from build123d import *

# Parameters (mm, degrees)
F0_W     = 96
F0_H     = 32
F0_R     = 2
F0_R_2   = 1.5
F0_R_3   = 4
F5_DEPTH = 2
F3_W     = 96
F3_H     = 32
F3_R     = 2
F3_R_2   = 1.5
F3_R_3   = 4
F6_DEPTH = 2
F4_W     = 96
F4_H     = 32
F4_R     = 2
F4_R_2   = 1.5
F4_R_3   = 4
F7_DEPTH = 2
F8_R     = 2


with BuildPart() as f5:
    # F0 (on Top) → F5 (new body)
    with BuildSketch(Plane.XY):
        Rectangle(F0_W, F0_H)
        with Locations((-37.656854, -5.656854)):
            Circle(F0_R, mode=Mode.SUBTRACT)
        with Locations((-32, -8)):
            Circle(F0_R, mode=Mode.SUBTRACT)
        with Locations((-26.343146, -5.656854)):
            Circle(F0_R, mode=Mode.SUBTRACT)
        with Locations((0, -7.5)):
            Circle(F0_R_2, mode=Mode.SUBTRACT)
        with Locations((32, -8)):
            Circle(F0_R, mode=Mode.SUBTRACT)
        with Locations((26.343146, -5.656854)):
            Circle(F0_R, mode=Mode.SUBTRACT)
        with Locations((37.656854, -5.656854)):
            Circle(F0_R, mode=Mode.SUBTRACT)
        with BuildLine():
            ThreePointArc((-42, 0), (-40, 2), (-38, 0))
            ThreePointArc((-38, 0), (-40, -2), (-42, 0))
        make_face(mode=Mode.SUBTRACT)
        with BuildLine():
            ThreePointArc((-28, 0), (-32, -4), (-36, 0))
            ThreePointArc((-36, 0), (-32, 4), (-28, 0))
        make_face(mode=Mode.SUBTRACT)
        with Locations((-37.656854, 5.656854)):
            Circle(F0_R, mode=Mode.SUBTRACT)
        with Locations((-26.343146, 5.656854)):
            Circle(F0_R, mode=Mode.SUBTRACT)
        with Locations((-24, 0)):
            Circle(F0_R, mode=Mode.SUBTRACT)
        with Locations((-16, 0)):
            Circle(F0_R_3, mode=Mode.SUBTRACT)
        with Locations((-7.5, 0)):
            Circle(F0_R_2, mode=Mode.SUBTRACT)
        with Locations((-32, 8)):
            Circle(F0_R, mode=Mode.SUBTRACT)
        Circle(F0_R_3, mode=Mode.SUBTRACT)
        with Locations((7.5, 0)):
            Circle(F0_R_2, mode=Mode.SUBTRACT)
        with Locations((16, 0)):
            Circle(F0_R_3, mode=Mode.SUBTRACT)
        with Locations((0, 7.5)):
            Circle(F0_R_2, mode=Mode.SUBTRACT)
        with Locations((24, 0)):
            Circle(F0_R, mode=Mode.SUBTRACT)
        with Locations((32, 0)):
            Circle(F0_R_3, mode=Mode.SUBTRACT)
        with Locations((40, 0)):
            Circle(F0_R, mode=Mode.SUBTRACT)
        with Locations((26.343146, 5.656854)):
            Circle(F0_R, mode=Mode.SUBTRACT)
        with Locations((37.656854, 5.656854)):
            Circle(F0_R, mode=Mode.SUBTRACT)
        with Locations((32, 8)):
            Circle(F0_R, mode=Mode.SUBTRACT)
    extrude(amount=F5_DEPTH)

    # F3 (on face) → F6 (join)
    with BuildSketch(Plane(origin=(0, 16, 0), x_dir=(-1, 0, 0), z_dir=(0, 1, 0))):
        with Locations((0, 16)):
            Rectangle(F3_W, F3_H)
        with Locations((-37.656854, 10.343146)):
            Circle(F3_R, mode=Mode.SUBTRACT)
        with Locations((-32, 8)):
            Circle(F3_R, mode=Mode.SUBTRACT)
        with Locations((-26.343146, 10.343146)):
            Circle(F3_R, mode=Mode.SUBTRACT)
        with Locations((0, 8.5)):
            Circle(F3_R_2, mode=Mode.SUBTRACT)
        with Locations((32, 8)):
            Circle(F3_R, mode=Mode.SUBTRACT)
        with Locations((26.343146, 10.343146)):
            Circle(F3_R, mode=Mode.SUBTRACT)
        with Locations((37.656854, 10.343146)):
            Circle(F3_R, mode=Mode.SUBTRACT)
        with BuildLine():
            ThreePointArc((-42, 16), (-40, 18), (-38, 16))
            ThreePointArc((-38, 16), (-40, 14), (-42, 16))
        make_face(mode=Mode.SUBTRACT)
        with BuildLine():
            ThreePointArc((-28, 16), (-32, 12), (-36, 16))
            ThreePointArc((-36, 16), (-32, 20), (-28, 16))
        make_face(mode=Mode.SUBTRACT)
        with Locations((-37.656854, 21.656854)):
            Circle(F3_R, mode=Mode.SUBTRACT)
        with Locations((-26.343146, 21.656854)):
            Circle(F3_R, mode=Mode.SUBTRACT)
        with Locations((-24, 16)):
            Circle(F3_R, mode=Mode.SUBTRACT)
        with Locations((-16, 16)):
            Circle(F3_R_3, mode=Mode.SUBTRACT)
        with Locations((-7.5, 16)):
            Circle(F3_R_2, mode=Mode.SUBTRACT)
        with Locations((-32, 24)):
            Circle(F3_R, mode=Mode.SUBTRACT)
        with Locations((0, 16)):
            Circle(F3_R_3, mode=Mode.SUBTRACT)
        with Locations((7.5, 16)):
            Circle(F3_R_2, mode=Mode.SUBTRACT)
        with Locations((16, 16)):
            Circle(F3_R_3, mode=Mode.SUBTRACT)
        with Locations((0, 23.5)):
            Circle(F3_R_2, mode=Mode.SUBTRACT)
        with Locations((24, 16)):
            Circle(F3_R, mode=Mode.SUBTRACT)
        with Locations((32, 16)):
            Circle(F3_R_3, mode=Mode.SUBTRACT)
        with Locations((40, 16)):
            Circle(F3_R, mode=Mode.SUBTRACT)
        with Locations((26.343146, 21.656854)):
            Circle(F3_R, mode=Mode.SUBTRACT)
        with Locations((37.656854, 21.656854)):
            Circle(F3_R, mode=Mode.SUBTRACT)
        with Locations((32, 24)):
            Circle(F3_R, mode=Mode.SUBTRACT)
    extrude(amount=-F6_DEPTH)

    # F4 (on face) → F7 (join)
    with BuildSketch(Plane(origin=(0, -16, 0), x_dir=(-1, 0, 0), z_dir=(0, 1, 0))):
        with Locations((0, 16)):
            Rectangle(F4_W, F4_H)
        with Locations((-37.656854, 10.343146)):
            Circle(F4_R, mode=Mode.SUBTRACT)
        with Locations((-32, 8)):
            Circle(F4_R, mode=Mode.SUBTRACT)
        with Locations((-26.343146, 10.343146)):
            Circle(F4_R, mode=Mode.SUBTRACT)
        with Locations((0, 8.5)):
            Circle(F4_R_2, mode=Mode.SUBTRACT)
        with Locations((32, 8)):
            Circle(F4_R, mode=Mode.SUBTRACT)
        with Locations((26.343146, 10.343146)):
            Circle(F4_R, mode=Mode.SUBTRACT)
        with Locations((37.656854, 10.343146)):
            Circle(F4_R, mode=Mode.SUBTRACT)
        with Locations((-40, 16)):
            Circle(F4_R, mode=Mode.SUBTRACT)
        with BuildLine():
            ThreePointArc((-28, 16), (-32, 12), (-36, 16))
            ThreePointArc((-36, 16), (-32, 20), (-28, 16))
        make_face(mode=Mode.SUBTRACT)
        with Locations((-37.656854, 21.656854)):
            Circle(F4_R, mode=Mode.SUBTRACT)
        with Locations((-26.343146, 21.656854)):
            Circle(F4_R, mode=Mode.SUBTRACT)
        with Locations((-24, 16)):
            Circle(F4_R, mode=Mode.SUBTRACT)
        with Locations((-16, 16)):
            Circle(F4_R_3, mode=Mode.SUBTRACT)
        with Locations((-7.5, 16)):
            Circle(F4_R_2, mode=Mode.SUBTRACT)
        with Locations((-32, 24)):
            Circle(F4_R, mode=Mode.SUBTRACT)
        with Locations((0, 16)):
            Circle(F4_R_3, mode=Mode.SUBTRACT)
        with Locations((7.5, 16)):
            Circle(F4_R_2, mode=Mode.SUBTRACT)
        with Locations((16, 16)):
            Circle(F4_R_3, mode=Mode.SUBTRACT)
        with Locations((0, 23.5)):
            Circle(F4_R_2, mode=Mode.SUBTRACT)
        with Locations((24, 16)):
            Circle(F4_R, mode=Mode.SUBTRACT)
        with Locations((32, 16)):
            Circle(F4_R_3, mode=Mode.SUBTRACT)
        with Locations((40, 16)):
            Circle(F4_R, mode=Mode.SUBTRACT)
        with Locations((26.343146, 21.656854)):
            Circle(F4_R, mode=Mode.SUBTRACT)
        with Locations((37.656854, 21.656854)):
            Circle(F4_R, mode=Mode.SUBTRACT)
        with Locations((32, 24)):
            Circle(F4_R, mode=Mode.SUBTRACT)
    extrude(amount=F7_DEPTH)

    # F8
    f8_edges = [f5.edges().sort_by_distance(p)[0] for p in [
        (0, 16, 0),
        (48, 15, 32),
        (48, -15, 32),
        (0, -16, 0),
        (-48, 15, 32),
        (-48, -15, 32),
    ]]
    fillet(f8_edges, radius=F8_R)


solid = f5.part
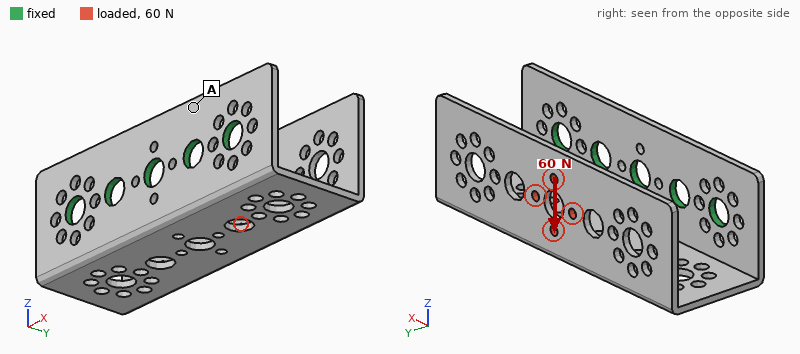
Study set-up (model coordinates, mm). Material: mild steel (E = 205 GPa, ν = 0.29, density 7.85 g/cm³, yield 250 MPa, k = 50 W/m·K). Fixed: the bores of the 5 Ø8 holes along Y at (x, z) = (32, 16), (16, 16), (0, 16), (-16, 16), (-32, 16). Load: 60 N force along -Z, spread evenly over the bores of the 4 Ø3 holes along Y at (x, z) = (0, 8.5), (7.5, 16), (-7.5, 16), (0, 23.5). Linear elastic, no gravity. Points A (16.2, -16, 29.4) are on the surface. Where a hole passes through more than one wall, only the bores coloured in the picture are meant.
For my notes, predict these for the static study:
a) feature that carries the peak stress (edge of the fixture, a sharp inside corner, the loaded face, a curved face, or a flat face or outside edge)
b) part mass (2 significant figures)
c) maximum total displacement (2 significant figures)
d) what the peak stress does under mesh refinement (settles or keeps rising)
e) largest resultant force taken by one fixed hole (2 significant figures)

a sharp inside corner
110 g
0.18 mm
keeps rising
23 N
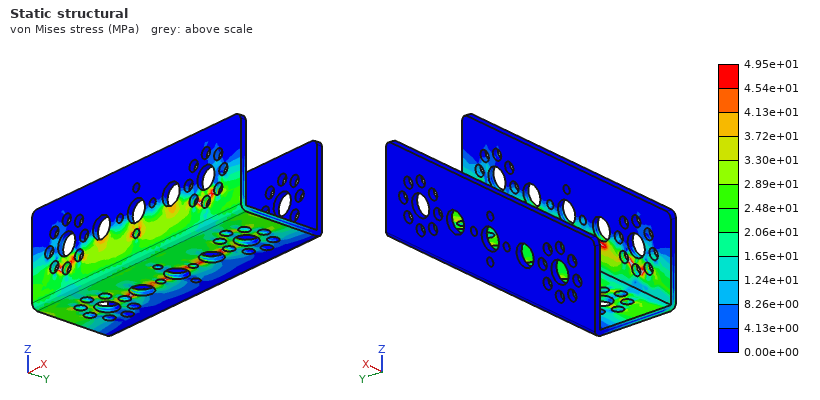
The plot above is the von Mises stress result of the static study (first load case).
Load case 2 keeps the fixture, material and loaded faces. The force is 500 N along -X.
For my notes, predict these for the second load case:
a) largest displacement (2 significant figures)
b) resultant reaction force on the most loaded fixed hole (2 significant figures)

0.46 mm
180 N
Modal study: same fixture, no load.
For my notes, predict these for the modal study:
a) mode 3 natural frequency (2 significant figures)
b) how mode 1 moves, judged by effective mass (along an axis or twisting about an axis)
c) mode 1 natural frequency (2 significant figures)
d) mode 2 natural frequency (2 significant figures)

1200 Hz
along Z
440 Hz
730 Hz
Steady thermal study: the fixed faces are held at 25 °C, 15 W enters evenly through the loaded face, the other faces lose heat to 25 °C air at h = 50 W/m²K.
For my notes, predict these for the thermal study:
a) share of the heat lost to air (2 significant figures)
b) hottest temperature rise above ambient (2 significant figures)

83 %
67 K
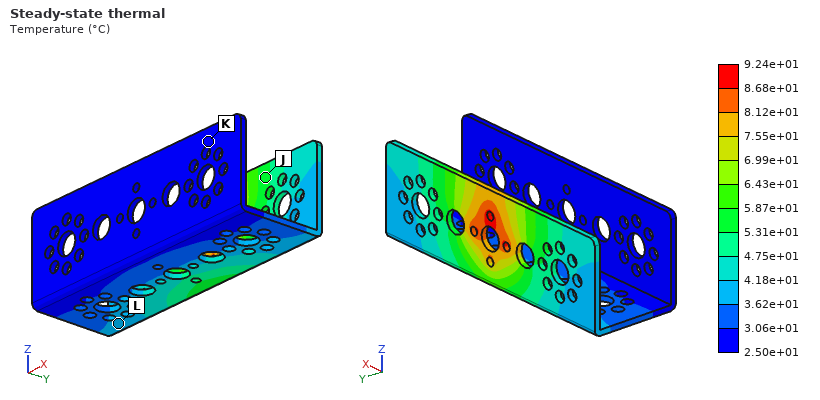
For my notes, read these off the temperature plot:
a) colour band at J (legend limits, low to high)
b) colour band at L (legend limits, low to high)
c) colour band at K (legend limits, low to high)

5.31e+01 to 5.87e+01 °C
3.62e+01 to 4.18e+01 °C
2.50e+01 to 3.06e+01 °C
